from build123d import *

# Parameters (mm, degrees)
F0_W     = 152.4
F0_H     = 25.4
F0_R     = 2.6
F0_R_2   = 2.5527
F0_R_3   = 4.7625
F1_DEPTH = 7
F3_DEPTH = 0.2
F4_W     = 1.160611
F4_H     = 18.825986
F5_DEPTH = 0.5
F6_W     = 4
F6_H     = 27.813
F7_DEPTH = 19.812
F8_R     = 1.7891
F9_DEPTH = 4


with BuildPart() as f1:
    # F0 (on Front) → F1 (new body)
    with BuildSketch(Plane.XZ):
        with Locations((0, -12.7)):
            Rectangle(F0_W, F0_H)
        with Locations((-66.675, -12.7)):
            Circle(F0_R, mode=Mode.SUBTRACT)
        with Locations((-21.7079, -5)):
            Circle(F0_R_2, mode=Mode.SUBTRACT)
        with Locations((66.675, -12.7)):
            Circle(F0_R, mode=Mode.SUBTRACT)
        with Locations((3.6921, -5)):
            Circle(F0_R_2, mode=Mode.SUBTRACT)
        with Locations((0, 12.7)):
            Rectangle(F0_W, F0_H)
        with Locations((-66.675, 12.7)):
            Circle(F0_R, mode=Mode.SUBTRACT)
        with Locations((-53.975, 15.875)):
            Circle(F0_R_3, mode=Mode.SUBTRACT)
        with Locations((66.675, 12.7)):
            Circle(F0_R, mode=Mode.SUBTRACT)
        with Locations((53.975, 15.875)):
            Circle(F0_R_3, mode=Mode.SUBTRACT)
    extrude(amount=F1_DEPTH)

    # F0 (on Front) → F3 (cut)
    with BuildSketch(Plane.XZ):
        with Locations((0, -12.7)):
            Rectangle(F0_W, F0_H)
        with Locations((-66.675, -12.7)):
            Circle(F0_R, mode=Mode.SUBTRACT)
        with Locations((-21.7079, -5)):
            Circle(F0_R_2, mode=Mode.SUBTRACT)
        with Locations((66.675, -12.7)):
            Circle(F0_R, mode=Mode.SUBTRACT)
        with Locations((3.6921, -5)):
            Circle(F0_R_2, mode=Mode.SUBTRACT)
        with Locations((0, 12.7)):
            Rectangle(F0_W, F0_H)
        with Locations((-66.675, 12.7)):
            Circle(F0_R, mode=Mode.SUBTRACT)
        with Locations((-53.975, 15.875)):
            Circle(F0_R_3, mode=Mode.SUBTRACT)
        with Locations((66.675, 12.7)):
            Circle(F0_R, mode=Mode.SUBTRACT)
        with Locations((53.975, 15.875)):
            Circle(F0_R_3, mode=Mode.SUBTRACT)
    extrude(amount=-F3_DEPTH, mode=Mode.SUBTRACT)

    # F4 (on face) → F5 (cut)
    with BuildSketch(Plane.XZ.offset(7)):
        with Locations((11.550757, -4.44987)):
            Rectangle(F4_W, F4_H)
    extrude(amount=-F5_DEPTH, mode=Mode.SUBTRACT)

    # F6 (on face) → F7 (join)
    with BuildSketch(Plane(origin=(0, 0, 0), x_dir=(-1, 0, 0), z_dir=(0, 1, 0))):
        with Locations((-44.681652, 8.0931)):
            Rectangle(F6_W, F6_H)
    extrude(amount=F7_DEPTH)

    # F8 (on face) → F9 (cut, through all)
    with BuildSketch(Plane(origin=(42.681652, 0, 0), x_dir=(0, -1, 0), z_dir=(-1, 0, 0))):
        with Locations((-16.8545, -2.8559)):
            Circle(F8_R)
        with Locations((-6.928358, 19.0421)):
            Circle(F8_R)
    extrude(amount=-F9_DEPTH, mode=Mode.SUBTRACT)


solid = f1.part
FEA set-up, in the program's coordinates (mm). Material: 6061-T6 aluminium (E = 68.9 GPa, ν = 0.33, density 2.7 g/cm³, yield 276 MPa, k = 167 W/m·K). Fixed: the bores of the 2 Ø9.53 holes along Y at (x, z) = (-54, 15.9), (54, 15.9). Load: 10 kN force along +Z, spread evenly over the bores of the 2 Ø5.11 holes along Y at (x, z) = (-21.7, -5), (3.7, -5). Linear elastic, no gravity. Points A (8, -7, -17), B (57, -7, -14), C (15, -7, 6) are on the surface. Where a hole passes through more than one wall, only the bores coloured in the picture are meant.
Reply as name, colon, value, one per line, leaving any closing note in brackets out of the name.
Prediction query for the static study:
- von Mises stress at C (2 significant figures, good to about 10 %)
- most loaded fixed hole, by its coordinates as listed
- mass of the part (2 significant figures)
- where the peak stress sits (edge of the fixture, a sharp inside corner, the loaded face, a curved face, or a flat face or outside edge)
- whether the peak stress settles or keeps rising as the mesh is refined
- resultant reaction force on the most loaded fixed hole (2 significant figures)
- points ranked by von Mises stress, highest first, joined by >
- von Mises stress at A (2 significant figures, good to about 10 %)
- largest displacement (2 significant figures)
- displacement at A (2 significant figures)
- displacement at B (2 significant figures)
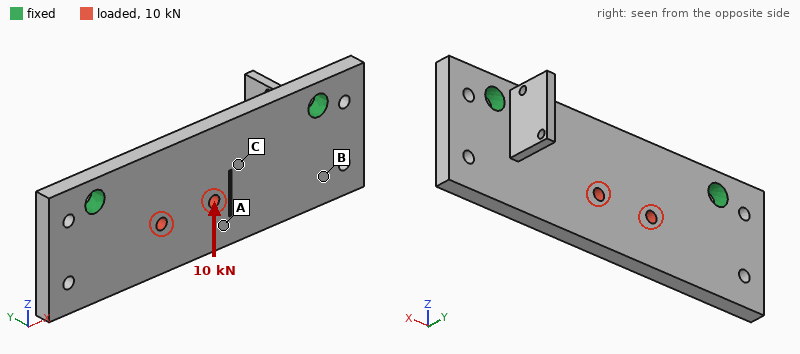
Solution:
von Mises stress at C: 27 MPa
most loaded fixed hole, by its coordinates as listed: (-54, 15.9)
mass of the part: 150 g
where the peak stress sits: edge of the fixture
whether the peak stress settles or keeps rising as the mesh is refined: keeps rising
resultant reaction force on the most loaded fixed hole: 6.8 kN
points ranked by von Mises stress, highest first, joined by >: A > C > B
von Mises stress at A: 38 MPa
largest displacement: 53 µm
displacement at A: 46 µm
displacement at B: 12 µm
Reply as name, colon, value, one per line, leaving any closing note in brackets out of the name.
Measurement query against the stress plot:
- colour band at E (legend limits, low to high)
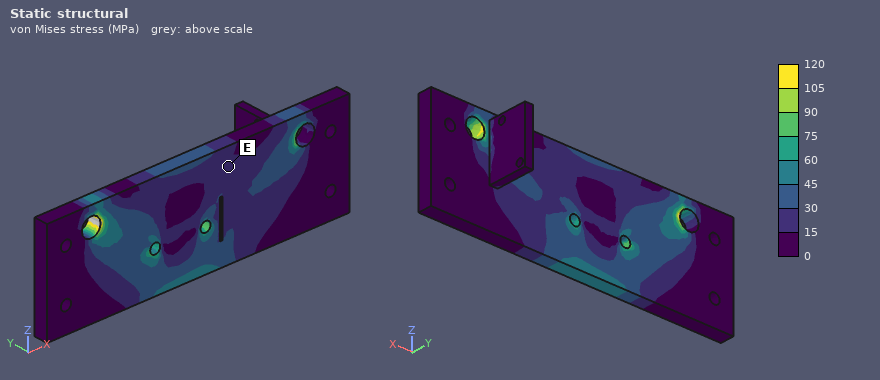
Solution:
colour band at E: 15 to 30 MPa
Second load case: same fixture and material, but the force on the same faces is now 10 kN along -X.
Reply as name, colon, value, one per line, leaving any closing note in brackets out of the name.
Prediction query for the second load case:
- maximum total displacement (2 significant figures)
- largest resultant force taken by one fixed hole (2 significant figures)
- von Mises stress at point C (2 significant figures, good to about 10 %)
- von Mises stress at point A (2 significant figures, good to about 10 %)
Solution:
maximum total displacement: 23 µm
largest resultant force taken by one fixed hole: 5.6 kN
von Mises stress at point C: 23 MPa
von Mises stress at point A: 7.9 MPa
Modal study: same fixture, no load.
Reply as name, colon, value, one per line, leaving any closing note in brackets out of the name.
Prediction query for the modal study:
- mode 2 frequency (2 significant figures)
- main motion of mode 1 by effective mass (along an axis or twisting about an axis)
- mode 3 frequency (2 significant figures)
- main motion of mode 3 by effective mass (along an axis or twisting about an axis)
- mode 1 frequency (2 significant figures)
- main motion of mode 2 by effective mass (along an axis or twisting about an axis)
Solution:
mode 2 frequency: 3600 Hz
main motion of mode 1 by effective mass: along Y
mode 3 frequency: 3900 Hz
main motion of mode 3 by effective mass: twisting about Z
mode 1 frequency: 2200 Hz
main motion of mode 2 by effective mass: twisting about X
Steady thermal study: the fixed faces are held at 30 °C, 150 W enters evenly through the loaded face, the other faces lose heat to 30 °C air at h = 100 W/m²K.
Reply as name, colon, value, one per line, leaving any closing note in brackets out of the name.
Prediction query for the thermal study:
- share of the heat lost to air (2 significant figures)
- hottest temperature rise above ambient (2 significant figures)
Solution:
share of the heat lost to air: 31 %
hottest temperature rise above ambient: 66 K
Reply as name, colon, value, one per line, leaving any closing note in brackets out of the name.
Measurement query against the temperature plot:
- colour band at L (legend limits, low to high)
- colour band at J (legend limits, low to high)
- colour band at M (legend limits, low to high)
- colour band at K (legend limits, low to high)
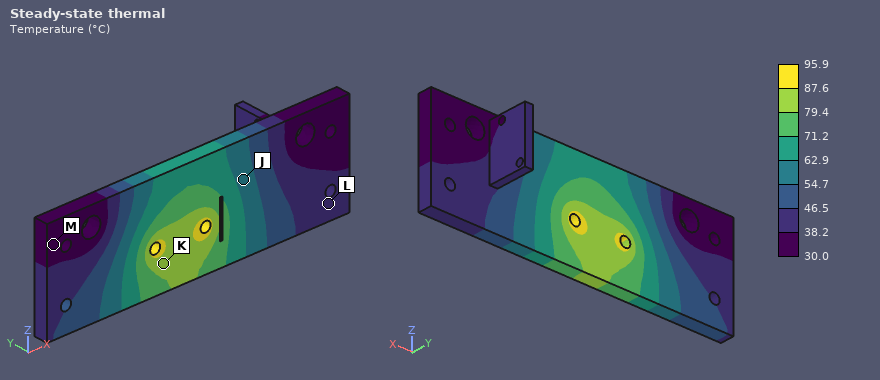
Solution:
colour band at L: 38.2 to 46.5 °C
colour band at J: 54.7 to 62.9 °C
colour band at M: 30.0 to 38.2 °C
colour band at K: 79.4 to 87.6 °C
